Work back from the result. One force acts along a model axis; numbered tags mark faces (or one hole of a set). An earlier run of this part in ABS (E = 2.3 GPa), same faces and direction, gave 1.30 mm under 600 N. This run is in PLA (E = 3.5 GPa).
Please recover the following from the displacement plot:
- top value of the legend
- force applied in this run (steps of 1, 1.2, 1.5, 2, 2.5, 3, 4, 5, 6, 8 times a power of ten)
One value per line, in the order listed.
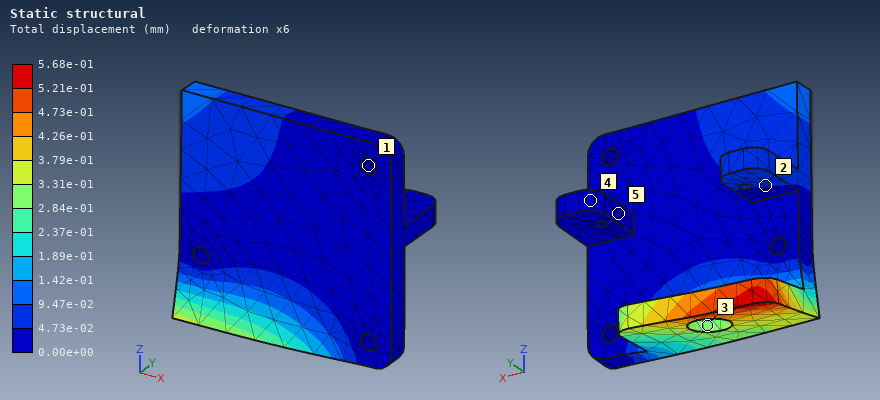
5.68e-01 mm
400 N
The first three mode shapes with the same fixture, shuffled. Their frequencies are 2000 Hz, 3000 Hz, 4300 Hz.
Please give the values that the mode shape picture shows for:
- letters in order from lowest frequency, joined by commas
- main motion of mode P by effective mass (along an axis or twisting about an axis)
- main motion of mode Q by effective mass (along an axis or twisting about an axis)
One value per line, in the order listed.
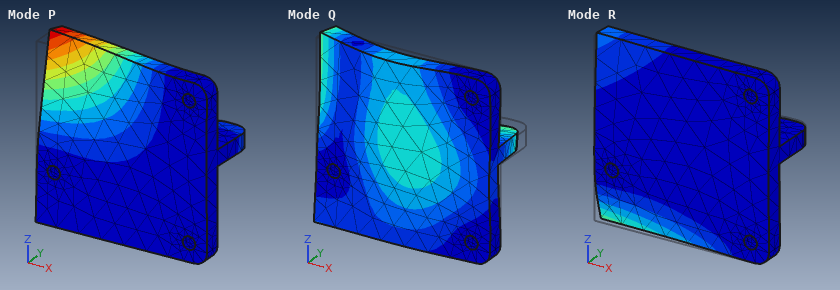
P, R, Q
along Y
along Y
